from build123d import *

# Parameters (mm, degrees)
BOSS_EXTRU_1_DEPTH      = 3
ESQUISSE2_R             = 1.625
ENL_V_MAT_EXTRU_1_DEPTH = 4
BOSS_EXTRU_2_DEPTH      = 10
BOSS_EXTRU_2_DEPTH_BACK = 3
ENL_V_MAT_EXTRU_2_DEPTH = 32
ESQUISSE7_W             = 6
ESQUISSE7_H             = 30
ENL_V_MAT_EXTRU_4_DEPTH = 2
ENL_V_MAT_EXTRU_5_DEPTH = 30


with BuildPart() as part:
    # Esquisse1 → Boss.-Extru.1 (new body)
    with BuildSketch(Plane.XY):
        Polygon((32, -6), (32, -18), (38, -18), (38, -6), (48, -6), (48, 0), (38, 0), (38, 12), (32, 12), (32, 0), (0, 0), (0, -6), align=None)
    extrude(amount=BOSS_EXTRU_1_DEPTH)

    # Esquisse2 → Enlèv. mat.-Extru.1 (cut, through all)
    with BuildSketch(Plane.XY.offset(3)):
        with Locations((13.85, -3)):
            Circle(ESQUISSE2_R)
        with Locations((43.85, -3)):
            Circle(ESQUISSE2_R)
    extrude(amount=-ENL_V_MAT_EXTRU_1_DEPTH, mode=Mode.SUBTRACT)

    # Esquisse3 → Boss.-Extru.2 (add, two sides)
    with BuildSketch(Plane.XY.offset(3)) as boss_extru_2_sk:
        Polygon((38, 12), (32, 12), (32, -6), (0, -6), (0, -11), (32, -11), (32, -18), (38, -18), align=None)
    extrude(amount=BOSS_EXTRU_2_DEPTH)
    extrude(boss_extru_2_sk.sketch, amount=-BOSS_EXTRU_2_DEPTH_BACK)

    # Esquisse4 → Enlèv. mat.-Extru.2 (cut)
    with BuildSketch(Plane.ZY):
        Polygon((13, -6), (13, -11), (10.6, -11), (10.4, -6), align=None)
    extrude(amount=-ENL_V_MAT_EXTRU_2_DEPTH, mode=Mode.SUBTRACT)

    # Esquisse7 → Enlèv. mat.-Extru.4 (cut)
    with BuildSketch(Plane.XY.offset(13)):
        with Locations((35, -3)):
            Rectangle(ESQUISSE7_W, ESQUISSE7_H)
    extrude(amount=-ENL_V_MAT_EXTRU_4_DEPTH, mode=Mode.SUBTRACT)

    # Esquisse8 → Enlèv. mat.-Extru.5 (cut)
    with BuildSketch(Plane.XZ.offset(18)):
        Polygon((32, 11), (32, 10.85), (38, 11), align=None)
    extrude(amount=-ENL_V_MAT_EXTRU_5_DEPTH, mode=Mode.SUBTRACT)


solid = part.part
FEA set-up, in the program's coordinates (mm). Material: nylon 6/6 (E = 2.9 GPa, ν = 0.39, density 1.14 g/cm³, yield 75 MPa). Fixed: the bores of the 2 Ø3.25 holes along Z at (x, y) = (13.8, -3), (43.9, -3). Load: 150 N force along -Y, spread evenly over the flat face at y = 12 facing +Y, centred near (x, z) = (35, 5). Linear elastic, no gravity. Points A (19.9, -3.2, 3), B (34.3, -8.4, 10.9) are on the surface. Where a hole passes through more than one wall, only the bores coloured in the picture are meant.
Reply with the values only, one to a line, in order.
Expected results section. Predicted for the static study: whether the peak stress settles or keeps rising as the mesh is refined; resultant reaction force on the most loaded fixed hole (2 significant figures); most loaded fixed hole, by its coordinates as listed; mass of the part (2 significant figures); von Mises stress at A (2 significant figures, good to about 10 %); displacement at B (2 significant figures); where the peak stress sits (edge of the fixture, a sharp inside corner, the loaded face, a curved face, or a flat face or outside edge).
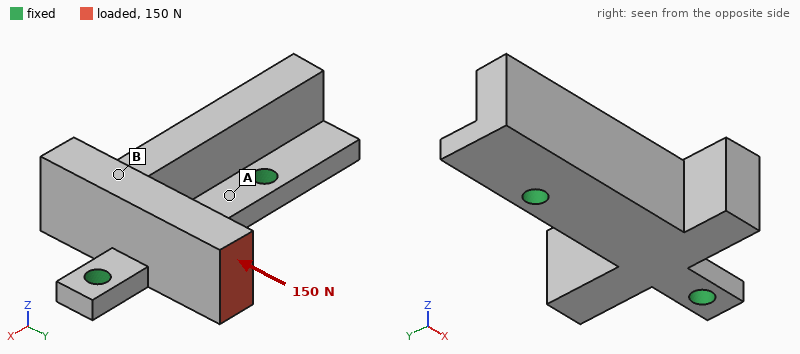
keeps rising
110 N
(43.9, -3)
5.0 g
11 MPa
0.33 mm
edge of the fixture
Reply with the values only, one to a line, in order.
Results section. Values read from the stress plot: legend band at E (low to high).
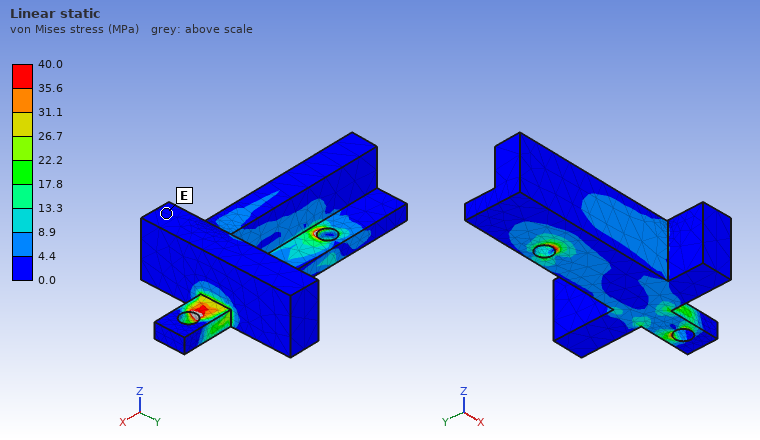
0.0 to 4.4 MPa
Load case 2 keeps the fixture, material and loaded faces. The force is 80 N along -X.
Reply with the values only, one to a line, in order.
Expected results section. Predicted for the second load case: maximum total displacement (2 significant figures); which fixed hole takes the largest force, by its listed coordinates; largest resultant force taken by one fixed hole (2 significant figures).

0.34 mm
(43.9, -3)
97 N
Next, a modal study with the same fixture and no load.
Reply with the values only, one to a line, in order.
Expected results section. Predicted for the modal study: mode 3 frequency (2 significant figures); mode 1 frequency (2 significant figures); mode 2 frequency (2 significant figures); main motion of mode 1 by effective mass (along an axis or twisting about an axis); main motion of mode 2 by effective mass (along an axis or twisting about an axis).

3900 Hz
1500 Hz
3500 Hz
along Y
along Z
